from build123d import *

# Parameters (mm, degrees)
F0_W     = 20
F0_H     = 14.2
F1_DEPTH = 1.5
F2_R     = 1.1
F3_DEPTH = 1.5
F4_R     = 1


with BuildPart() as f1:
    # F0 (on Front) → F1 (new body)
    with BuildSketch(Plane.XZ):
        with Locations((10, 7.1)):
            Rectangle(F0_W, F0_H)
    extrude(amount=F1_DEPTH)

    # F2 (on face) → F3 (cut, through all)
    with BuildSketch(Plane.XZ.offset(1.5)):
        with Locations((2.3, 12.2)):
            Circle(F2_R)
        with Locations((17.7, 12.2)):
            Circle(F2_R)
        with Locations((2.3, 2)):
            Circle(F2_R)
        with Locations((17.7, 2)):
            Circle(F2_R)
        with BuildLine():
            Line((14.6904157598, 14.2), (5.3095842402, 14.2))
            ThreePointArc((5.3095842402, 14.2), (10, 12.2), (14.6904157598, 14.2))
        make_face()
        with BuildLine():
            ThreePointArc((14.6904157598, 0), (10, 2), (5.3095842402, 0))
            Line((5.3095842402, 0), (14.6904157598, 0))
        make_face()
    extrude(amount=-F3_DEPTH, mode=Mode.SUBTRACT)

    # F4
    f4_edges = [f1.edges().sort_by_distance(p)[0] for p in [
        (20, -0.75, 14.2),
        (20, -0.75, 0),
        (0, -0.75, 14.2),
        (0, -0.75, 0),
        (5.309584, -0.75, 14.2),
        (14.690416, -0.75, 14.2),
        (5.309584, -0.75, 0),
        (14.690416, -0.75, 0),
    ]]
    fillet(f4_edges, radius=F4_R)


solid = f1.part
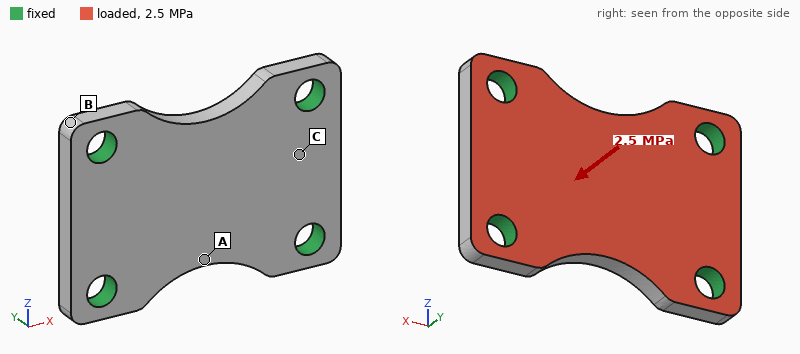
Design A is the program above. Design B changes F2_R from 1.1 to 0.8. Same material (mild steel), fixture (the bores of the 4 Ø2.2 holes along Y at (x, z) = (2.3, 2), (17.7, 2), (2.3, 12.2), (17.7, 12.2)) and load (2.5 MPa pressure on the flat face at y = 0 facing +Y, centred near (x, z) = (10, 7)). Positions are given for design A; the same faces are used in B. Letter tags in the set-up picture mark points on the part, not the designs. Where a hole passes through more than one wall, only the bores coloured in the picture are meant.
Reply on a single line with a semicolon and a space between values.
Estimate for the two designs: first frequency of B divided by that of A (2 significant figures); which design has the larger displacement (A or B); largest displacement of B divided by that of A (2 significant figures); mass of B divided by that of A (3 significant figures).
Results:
0.90; B; 1.2; 1.03
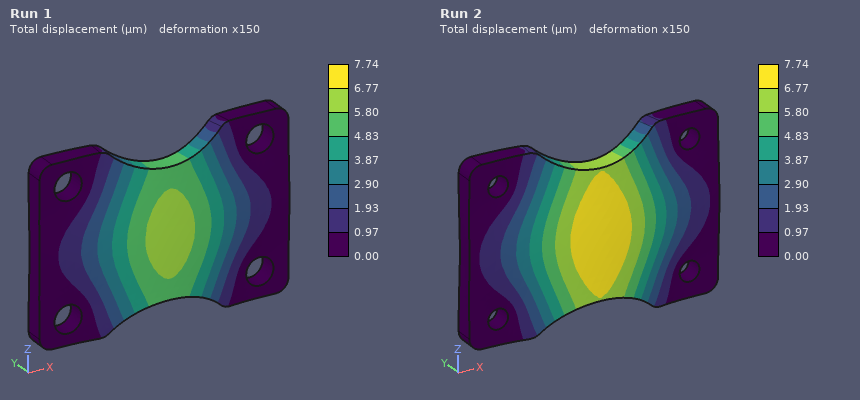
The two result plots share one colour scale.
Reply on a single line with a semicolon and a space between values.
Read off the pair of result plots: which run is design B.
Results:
Run 2
